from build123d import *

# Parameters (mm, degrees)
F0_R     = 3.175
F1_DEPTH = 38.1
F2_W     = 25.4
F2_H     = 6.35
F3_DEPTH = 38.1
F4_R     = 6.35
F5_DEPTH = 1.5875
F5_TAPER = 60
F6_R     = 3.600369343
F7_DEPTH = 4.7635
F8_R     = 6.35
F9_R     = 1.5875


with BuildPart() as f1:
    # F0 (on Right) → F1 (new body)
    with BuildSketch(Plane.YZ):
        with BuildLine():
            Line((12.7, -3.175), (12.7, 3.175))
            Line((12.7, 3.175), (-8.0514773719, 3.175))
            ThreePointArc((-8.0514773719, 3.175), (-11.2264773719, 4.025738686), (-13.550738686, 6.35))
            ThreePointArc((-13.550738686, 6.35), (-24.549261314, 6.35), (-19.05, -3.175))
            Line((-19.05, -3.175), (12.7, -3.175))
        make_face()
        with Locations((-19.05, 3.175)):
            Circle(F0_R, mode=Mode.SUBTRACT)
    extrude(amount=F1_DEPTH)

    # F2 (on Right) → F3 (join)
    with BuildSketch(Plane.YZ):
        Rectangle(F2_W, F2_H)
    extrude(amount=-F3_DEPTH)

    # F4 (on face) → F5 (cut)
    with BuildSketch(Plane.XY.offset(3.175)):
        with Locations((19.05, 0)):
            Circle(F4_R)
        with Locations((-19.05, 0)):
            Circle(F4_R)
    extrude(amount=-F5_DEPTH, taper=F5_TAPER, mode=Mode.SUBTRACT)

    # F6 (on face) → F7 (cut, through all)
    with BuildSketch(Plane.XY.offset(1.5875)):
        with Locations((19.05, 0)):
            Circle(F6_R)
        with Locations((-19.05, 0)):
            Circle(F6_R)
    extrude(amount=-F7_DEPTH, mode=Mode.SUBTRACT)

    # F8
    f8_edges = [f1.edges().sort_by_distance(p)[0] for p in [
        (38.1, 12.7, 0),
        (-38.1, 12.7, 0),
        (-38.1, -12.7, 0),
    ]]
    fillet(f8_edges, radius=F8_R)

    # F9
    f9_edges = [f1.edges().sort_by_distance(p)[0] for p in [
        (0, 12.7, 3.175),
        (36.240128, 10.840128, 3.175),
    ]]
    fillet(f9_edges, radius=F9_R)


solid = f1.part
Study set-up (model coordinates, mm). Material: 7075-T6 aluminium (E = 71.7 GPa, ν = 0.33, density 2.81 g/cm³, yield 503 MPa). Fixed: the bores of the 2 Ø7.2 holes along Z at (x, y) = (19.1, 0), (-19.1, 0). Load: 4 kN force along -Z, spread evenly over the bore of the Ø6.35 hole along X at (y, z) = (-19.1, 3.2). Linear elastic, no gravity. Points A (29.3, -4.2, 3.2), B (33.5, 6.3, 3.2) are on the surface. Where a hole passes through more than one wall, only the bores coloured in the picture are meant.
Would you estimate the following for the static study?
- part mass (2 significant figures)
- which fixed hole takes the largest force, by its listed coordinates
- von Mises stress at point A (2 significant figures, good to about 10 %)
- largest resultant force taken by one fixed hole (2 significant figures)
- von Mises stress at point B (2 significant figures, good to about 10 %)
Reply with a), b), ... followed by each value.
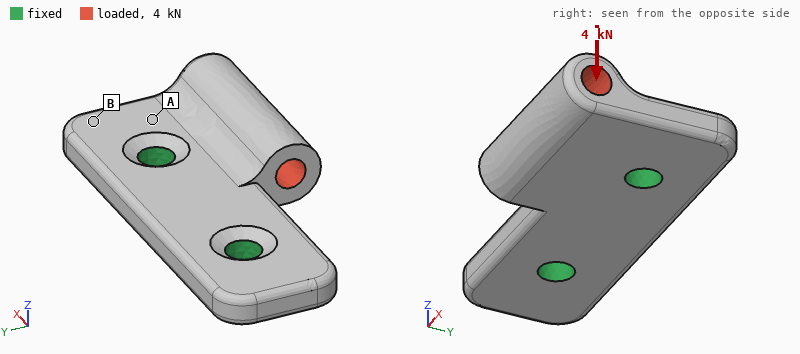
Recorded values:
a) 43 g
b) (19.1, 0)
c) 150 MPa
d) 3.8 kN
e) 50 MPa
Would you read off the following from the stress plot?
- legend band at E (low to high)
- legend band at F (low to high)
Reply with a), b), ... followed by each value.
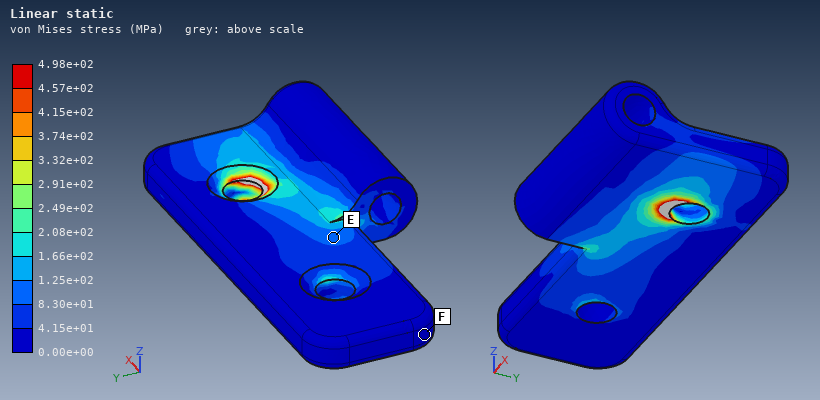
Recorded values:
a) 8.30e+01 to 1.25e+02 MPa
b) 0.00e+00 to 4.15e+01 MPa
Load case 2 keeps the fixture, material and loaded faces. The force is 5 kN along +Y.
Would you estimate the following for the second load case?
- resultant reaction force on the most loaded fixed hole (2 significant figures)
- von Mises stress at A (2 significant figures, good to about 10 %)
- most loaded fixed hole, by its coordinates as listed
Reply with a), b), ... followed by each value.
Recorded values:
a) 4.8 kN
b) 62 MPa
c) (19.1, 0)
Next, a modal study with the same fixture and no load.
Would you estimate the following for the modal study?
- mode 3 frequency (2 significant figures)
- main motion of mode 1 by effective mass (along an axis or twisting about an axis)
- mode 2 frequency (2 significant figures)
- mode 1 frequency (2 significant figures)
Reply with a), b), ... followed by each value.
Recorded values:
a) 14 kHz
b) along Z
c) 10 kHz
d) 6200 Hz
